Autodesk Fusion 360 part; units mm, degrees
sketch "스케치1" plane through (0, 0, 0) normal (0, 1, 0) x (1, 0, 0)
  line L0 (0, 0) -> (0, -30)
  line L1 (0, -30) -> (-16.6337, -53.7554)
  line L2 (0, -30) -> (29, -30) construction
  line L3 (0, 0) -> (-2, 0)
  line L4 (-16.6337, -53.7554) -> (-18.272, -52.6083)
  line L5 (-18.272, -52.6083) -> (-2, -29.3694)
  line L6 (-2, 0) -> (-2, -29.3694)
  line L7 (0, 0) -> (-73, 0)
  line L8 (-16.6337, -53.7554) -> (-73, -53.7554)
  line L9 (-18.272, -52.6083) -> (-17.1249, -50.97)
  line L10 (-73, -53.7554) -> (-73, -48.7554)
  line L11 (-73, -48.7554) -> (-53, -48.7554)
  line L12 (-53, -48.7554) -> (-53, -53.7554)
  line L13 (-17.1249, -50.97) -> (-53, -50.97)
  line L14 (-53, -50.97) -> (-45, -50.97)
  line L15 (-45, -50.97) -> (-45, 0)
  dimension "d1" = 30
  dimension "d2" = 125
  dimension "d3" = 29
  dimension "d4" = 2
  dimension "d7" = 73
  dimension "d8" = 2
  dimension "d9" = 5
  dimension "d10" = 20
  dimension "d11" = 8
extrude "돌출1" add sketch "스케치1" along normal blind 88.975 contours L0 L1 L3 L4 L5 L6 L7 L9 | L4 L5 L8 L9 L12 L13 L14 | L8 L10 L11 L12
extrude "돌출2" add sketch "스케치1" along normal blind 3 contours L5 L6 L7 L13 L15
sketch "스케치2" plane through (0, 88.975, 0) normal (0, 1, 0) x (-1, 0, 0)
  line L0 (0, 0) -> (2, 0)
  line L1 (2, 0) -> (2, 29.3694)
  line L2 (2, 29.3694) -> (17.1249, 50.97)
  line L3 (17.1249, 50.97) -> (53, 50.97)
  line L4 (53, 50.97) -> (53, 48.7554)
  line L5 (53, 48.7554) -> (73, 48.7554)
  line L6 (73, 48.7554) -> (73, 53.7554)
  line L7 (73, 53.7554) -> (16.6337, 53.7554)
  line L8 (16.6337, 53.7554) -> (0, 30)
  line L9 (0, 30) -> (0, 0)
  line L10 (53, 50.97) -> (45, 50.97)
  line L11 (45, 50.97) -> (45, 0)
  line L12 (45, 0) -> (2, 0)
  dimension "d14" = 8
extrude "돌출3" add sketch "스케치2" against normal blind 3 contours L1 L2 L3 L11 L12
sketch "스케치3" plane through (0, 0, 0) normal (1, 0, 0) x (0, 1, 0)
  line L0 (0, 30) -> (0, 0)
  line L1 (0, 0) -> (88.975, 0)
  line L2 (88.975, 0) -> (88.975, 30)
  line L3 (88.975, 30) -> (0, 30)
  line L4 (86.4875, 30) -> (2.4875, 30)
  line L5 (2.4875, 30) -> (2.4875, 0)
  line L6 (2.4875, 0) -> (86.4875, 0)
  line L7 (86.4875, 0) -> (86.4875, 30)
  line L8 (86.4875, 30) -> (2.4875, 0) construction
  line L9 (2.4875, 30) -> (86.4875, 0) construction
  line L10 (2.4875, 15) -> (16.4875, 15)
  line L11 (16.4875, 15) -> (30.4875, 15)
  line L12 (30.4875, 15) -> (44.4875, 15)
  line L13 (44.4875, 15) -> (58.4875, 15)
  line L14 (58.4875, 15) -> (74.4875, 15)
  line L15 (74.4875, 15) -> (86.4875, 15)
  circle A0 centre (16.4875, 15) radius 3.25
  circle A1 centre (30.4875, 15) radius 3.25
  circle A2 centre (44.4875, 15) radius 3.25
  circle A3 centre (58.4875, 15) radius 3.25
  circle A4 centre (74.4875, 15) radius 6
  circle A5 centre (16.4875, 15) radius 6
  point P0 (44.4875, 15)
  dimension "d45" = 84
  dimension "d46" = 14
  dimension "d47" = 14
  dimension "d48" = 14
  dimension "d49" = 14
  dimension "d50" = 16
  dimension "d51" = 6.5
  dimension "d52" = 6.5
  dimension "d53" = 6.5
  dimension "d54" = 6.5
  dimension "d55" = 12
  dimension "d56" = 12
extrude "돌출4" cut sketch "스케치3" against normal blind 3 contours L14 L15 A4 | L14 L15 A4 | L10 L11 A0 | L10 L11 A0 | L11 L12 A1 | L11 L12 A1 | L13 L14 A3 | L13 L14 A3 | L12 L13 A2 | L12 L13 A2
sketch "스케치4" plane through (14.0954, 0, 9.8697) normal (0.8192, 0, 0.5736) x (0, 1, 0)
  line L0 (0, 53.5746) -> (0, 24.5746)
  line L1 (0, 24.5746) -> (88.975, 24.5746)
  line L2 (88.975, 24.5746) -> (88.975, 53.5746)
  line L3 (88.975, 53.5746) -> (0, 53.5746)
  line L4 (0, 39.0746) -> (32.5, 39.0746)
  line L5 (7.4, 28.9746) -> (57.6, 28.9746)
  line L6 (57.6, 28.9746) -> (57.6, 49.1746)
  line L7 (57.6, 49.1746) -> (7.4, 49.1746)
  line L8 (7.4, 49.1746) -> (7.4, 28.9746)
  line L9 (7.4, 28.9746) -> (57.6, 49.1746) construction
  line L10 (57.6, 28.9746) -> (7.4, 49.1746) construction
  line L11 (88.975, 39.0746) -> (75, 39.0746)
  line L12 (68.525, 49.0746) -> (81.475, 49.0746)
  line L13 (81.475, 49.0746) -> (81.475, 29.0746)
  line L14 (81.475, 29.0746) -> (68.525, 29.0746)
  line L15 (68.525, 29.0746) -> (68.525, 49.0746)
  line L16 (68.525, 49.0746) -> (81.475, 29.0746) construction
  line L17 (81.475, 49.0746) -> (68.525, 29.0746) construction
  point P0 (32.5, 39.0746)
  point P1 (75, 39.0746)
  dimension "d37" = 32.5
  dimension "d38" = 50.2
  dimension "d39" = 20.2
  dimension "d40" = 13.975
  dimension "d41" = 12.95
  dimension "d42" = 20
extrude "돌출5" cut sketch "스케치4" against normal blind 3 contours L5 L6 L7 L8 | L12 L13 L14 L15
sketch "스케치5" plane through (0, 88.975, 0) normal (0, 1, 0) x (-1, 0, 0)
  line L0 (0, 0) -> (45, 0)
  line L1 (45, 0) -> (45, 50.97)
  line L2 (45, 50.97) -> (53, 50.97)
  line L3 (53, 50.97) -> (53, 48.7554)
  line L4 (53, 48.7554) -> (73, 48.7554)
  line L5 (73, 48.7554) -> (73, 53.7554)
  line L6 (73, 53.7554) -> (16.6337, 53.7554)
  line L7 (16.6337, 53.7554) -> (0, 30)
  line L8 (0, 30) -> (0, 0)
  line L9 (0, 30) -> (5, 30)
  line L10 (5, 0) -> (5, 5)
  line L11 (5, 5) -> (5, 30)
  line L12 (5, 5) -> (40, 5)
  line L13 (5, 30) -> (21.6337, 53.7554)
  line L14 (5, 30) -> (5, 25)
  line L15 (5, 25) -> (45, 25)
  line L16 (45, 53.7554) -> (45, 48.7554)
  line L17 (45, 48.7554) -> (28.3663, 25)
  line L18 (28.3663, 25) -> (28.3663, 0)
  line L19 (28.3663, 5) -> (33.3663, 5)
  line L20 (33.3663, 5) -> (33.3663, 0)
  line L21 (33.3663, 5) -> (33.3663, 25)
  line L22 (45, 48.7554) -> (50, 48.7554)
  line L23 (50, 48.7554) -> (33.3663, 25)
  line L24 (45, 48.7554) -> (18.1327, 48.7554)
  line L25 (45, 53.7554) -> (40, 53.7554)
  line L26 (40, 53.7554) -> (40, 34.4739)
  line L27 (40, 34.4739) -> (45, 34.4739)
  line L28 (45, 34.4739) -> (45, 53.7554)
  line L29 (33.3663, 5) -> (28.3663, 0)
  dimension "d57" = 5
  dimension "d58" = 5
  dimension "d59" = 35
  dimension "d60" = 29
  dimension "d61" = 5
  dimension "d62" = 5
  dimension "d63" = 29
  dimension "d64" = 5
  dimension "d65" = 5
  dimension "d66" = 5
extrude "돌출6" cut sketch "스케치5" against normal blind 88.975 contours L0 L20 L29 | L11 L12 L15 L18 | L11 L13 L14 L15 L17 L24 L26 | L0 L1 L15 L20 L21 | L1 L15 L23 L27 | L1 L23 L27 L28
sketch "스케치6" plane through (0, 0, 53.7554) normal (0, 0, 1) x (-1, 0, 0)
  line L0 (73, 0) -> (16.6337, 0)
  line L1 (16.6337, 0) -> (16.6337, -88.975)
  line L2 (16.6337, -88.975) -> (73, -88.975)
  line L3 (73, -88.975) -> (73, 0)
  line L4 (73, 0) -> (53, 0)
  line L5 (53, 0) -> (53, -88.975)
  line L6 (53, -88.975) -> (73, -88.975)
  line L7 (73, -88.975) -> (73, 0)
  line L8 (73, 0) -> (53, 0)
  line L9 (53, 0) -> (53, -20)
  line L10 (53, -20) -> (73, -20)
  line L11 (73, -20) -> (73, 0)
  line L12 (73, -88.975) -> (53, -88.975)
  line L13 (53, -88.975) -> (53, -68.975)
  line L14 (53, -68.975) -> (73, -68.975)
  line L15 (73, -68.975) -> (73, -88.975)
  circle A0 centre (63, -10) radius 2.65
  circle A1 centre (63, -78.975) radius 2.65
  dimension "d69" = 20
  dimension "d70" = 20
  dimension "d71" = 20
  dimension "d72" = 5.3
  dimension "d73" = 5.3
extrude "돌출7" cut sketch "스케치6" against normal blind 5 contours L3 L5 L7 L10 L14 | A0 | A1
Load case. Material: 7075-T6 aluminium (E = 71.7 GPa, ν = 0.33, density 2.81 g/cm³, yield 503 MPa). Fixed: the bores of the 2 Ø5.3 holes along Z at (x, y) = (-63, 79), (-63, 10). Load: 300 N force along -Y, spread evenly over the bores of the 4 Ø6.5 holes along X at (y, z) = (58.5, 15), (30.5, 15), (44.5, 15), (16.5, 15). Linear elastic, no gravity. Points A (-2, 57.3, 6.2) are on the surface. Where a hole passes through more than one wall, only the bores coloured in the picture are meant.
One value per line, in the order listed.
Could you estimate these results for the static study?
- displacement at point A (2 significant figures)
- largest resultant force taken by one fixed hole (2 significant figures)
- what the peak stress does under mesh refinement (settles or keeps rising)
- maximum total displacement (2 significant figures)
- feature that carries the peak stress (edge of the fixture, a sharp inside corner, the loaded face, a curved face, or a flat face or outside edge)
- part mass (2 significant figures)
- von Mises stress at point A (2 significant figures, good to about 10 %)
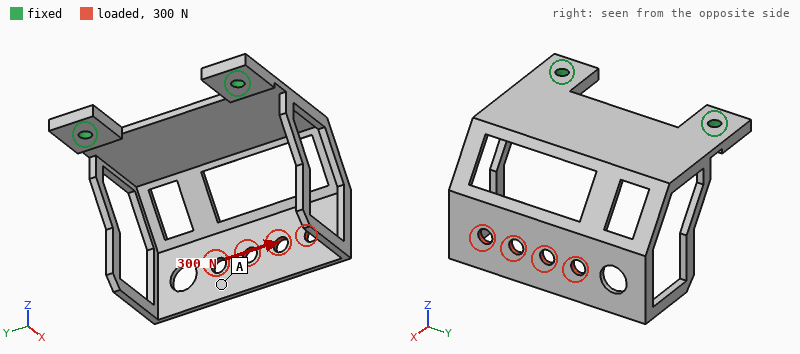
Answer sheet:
0.72 mm
320 N
keeps rising
1.2 mm
a sharp inside corner
65 g
34 MPa
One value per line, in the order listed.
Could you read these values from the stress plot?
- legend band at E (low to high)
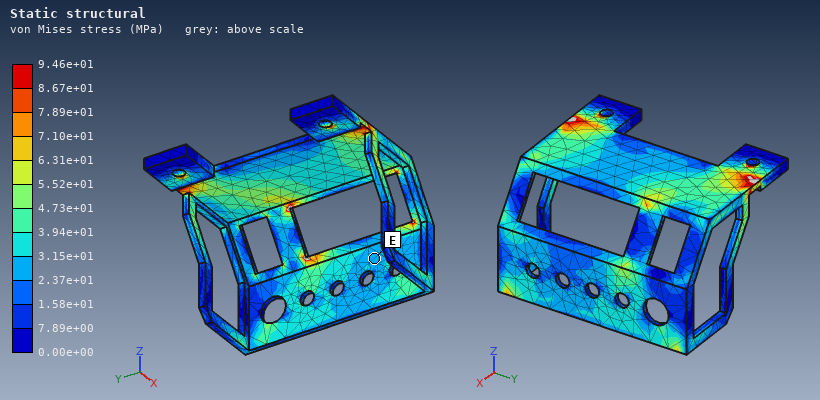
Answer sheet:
2.37e+01 to 3.15e+01 MPa
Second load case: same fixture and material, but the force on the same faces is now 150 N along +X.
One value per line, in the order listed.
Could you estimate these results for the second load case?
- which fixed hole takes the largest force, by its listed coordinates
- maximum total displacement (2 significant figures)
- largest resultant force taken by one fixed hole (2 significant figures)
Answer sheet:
(-63, 10)
1.5 mm
97 N
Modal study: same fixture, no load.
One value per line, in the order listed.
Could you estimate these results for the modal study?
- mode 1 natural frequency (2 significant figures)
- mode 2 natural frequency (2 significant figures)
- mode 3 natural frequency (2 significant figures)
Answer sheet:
320 Hz
510 Hz
1200 Hz
